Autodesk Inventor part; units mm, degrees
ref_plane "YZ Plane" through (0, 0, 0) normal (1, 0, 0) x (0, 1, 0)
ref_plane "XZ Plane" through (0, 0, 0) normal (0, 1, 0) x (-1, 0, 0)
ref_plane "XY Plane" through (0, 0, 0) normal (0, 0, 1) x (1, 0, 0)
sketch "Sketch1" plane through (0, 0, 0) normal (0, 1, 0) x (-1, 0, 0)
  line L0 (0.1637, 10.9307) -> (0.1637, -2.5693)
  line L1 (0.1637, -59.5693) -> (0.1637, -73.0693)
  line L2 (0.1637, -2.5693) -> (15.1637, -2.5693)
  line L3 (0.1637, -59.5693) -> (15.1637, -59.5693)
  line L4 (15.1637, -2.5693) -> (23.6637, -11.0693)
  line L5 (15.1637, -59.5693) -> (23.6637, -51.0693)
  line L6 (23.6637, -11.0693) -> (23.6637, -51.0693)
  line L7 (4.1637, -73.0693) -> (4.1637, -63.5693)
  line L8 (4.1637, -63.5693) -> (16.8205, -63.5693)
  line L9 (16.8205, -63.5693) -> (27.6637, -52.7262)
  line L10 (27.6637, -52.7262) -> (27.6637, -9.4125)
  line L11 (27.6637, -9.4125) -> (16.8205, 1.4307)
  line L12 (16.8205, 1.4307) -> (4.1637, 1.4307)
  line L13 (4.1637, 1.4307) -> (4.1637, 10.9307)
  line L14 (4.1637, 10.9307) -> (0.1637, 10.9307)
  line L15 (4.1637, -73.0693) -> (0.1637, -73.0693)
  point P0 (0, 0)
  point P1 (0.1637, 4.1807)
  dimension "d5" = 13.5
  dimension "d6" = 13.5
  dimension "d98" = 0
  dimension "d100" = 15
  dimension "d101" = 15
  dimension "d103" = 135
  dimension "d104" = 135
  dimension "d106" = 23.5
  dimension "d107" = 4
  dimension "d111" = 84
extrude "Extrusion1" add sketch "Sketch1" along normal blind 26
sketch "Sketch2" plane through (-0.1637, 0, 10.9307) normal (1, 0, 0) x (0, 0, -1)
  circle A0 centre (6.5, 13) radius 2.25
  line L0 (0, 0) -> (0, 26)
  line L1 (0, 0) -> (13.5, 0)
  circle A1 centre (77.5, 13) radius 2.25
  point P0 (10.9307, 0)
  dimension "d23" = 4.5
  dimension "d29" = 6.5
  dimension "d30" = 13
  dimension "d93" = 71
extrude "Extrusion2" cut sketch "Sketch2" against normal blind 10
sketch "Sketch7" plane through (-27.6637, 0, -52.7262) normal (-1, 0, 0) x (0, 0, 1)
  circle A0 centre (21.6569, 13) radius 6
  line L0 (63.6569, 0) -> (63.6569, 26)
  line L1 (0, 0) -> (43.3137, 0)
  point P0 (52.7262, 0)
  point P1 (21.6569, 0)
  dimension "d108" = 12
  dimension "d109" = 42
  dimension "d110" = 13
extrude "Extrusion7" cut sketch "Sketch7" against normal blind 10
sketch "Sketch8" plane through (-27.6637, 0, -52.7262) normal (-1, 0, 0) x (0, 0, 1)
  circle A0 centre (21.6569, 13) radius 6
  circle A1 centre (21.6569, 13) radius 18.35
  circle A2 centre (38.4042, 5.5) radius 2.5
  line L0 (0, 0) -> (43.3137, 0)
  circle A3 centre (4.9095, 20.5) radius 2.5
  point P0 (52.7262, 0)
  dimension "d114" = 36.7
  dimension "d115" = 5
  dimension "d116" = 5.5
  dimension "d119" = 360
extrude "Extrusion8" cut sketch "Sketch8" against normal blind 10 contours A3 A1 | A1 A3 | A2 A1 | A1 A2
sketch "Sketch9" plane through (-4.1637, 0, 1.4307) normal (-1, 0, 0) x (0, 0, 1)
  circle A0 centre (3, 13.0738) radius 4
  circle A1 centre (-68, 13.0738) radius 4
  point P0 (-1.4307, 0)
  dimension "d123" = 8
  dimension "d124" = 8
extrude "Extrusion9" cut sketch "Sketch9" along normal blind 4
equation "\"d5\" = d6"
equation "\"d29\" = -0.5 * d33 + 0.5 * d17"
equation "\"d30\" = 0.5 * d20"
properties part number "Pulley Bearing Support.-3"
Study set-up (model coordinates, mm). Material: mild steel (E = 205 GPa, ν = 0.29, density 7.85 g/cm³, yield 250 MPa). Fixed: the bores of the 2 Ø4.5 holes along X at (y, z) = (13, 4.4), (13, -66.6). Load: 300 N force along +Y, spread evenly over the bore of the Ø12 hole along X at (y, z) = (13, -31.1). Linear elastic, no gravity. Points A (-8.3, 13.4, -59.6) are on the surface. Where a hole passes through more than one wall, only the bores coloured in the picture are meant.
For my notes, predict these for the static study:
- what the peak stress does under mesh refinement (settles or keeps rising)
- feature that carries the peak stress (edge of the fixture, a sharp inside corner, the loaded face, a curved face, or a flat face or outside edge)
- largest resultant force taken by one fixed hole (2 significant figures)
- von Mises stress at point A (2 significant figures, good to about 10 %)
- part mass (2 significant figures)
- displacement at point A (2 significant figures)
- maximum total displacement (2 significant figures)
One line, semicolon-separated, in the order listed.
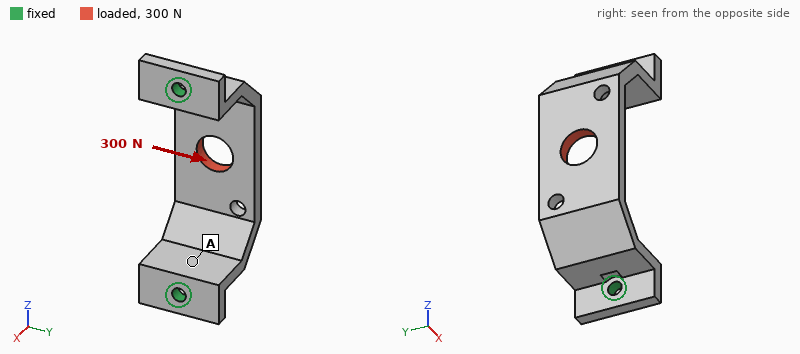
keeps rising; edge of the fixture; 150 N; 9.0 MPa; 92 g; 2.9 µm; 14 µm
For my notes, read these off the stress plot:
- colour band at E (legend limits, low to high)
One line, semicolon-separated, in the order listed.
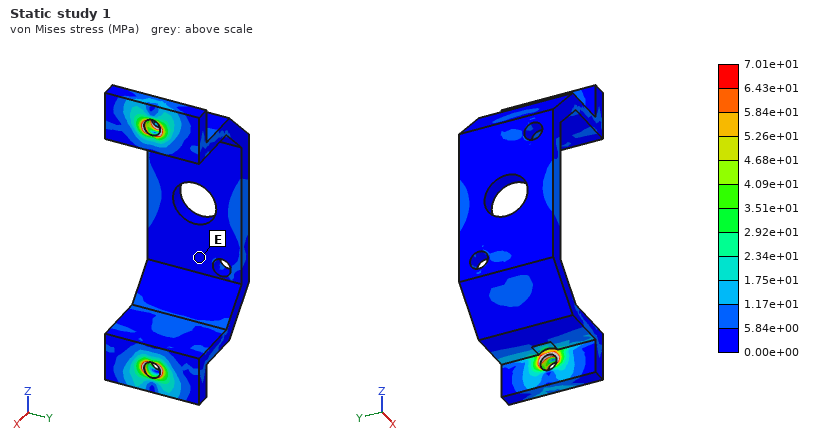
0.00e+00 to 5.84e+00 MPa
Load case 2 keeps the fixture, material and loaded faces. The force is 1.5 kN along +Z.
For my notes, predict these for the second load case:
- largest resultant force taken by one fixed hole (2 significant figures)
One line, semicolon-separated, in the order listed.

810 N
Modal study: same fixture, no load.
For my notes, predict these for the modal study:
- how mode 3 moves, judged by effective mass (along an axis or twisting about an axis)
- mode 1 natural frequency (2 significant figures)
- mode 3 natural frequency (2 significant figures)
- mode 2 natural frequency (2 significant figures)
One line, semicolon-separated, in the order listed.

twisting about X; 3600 Hz; 5800 Hz; 3700 Hz
